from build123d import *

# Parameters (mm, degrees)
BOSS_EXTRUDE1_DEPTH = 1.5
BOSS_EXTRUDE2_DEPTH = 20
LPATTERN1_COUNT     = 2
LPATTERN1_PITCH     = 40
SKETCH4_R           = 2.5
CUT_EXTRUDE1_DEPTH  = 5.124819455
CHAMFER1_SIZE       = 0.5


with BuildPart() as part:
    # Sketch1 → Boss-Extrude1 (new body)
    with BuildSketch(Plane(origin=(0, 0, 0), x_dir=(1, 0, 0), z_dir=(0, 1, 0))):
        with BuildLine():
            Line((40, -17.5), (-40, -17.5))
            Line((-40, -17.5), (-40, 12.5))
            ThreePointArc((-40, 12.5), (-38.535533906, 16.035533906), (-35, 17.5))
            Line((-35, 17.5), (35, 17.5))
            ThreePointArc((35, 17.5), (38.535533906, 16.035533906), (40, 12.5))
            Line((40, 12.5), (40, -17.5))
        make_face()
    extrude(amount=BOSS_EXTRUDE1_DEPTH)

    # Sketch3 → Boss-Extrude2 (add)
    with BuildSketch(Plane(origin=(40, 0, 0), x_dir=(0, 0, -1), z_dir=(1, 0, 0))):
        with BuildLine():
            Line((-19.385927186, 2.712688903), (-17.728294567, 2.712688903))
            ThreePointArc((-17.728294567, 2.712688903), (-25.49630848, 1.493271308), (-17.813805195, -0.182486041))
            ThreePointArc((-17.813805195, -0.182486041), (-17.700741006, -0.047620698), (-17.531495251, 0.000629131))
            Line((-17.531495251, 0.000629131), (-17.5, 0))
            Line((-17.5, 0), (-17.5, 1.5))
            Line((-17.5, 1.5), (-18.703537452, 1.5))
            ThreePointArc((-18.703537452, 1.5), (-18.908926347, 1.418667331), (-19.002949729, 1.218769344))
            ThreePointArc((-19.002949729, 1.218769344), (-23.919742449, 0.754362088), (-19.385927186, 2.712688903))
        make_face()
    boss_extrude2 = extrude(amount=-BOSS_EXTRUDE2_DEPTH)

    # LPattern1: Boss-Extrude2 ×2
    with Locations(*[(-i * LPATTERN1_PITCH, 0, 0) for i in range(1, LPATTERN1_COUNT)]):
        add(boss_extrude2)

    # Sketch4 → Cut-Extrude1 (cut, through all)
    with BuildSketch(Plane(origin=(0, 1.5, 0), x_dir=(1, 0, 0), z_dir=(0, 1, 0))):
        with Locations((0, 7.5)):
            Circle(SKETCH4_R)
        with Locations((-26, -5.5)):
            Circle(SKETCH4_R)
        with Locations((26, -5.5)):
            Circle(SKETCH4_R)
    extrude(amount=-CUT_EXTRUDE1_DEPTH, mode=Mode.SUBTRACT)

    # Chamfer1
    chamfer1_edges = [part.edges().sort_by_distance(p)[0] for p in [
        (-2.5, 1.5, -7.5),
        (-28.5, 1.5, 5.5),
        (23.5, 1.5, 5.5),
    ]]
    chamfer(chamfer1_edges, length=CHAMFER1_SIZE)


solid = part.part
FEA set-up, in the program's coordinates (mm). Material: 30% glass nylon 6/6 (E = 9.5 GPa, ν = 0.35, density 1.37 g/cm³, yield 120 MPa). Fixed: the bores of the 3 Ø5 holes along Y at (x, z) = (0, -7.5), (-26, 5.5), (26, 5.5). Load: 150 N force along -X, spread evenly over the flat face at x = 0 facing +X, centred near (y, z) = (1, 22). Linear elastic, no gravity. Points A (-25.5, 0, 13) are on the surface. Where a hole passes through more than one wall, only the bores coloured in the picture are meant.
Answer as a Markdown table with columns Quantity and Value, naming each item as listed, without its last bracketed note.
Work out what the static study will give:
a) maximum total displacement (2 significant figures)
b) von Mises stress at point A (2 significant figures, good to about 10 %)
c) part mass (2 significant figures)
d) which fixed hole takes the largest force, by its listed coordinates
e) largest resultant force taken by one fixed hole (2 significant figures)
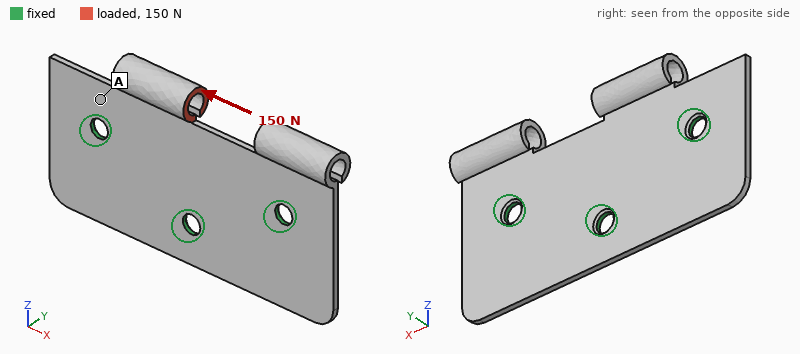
| Quantity | Value |
|---|---|
| maximum total displacement | 0.44 mm |
| von Mises stress at point A | 7.9 MPa |
| part mass | 7.2 g |
| which fixed hole takes the largest force, by its listed coordinates | (-26, 5.5) |
| largest resultant force taken by one fixed hole | 110 N |
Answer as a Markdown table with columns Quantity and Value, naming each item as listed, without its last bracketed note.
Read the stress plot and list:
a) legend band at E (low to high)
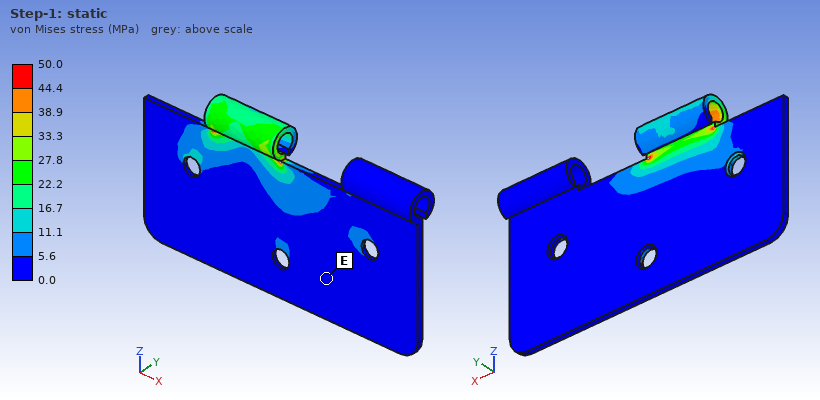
| Quantity | Value |
|---|---|
| legend band at E | 0.0 to 5.6 MPa |
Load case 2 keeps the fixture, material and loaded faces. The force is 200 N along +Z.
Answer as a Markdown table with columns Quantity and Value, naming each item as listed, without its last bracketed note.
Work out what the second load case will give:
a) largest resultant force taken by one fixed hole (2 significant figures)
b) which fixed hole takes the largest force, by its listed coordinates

| Quantity | Value |
|---|---|
| largest resultant force taken by one fixed hole | 150 N |
| which fixed hole takes the largest force, by its listed coordinates | (0, -7.5) |
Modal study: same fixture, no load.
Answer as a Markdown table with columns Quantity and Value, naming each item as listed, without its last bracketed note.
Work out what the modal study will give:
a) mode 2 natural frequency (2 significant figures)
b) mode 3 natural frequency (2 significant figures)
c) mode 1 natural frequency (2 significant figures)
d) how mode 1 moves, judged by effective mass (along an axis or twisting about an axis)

| Quantity | Value |
|---|---|
| mode 2 natural frequency | 1100 Hz |
| mode 3 natural frequency | 1600 Hz |
| mode 1 natural frequency | 1000 Hz |
| how mode 1 moves, judged by effective mass | along Y |
